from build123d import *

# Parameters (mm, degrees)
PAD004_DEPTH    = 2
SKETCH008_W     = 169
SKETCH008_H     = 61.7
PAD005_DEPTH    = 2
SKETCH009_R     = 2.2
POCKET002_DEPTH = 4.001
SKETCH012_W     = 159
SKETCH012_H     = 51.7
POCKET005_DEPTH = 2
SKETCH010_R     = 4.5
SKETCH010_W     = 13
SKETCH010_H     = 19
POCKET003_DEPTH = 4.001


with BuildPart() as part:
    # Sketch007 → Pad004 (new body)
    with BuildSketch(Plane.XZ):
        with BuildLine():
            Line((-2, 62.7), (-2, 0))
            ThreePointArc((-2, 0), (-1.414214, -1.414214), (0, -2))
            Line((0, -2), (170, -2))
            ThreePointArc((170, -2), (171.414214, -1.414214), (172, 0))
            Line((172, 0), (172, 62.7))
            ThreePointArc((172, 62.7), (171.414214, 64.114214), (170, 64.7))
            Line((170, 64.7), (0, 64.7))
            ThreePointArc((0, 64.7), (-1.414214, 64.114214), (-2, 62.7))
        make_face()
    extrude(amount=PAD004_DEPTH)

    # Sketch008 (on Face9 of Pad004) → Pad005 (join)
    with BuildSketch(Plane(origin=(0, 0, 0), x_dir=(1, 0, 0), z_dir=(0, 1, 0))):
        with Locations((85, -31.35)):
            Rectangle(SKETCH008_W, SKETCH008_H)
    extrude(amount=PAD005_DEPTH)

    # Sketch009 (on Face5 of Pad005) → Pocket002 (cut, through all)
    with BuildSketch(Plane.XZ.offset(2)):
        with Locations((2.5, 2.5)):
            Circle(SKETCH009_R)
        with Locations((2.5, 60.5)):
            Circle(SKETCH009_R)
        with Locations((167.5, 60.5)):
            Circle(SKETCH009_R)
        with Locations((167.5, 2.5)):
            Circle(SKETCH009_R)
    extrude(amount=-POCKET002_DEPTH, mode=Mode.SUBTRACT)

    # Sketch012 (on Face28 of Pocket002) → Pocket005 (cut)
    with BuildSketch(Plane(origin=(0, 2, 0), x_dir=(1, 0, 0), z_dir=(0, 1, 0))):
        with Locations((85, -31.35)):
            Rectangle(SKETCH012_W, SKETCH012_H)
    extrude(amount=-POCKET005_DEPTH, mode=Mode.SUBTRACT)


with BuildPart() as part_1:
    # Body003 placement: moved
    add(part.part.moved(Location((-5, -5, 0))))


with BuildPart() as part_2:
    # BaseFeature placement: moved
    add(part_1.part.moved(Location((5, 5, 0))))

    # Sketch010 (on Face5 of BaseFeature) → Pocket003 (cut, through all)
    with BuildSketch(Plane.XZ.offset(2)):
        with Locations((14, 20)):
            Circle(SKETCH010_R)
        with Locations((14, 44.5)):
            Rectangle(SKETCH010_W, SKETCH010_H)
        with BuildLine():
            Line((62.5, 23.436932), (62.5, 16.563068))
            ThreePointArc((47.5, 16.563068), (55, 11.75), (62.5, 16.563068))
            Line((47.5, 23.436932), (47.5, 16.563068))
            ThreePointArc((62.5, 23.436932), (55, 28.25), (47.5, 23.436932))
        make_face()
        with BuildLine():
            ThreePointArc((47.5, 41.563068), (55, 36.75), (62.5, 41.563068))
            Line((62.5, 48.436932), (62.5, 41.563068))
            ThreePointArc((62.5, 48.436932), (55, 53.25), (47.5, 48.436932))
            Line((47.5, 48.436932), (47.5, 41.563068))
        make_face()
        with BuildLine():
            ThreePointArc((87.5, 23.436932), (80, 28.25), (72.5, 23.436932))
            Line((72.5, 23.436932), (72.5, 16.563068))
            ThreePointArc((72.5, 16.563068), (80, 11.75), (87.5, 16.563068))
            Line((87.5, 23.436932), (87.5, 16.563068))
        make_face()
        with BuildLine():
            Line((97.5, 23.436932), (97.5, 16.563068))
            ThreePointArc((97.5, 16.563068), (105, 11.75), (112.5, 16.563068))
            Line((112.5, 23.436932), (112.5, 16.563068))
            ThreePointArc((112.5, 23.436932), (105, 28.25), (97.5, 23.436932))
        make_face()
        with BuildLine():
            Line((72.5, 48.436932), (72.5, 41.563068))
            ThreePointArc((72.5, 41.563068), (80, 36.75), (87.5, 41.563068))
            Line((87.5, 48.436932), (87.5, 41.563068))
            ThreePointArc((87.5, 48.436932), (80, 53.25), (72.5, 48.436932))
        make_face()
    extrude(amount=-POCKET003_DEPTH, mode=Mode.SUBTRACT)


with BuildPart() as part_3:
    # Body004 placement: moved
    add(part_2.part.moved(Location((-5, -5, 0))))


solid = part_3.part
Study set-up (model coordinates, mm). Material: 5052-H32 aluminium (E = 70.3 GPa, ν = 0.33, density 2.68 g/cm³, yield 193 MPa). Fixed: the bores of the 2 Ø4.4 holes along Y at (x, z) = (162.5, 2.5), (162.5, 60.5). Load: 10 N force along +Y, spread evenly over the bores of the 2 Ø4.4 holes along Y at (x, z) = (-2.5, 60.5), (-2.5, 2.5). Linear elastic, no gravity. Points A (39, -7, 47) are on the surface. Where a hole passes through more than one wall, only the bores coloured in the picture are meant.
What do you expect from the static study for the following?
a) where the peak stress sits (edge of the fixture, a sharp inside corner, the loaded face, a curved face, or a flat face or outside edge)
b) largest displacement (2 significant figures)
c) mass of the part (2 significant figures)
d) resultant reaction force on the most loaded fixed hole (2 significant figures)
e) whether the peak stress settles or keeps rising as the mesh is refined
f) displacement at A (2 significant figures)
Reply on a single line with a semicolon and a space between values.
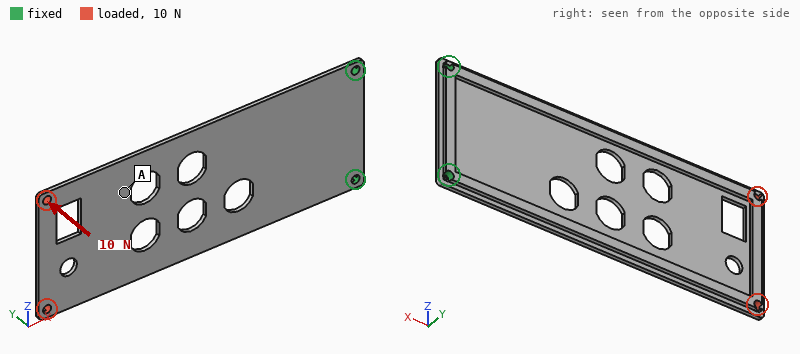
edge of the fixture; 2.0 mm; 66 g; 47 N; keeps rising; 1.2 mm
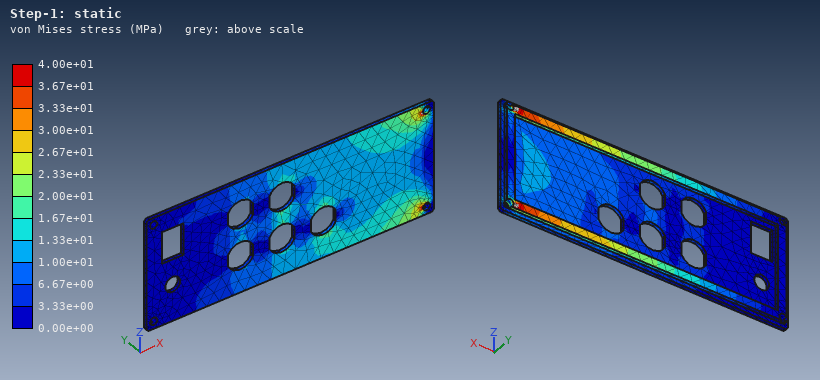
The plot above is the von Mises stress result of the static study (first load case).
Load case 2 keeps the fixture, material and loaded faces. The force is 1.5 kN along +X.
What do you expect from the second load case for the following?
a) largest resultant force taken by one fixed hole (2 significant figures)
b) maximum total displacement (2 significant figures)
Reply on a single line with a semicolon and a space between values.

790 N; 1.2 mm
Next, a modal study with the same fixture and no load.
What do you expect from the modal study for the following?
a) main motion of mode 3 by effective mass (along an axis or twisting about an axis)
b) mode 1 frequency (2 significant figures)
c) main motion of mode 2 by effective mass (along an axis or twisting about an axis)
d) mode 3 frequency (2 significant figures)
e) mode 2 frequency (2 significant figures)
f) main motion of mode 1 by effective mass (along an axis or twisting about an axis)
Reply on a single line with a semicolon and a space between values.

along Y; 89 Hz; twisting about X; 540 Hz; 360 Hz; along Y
